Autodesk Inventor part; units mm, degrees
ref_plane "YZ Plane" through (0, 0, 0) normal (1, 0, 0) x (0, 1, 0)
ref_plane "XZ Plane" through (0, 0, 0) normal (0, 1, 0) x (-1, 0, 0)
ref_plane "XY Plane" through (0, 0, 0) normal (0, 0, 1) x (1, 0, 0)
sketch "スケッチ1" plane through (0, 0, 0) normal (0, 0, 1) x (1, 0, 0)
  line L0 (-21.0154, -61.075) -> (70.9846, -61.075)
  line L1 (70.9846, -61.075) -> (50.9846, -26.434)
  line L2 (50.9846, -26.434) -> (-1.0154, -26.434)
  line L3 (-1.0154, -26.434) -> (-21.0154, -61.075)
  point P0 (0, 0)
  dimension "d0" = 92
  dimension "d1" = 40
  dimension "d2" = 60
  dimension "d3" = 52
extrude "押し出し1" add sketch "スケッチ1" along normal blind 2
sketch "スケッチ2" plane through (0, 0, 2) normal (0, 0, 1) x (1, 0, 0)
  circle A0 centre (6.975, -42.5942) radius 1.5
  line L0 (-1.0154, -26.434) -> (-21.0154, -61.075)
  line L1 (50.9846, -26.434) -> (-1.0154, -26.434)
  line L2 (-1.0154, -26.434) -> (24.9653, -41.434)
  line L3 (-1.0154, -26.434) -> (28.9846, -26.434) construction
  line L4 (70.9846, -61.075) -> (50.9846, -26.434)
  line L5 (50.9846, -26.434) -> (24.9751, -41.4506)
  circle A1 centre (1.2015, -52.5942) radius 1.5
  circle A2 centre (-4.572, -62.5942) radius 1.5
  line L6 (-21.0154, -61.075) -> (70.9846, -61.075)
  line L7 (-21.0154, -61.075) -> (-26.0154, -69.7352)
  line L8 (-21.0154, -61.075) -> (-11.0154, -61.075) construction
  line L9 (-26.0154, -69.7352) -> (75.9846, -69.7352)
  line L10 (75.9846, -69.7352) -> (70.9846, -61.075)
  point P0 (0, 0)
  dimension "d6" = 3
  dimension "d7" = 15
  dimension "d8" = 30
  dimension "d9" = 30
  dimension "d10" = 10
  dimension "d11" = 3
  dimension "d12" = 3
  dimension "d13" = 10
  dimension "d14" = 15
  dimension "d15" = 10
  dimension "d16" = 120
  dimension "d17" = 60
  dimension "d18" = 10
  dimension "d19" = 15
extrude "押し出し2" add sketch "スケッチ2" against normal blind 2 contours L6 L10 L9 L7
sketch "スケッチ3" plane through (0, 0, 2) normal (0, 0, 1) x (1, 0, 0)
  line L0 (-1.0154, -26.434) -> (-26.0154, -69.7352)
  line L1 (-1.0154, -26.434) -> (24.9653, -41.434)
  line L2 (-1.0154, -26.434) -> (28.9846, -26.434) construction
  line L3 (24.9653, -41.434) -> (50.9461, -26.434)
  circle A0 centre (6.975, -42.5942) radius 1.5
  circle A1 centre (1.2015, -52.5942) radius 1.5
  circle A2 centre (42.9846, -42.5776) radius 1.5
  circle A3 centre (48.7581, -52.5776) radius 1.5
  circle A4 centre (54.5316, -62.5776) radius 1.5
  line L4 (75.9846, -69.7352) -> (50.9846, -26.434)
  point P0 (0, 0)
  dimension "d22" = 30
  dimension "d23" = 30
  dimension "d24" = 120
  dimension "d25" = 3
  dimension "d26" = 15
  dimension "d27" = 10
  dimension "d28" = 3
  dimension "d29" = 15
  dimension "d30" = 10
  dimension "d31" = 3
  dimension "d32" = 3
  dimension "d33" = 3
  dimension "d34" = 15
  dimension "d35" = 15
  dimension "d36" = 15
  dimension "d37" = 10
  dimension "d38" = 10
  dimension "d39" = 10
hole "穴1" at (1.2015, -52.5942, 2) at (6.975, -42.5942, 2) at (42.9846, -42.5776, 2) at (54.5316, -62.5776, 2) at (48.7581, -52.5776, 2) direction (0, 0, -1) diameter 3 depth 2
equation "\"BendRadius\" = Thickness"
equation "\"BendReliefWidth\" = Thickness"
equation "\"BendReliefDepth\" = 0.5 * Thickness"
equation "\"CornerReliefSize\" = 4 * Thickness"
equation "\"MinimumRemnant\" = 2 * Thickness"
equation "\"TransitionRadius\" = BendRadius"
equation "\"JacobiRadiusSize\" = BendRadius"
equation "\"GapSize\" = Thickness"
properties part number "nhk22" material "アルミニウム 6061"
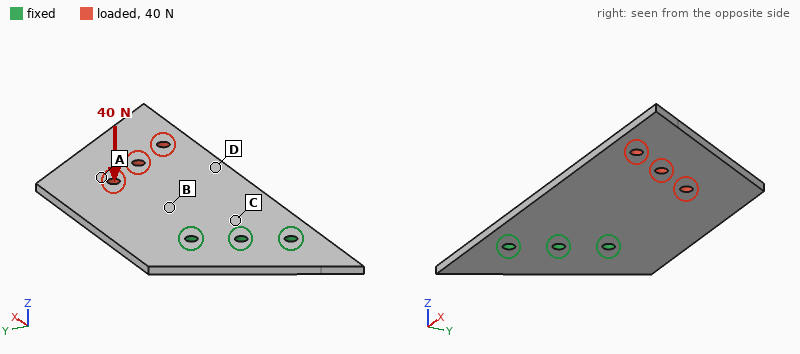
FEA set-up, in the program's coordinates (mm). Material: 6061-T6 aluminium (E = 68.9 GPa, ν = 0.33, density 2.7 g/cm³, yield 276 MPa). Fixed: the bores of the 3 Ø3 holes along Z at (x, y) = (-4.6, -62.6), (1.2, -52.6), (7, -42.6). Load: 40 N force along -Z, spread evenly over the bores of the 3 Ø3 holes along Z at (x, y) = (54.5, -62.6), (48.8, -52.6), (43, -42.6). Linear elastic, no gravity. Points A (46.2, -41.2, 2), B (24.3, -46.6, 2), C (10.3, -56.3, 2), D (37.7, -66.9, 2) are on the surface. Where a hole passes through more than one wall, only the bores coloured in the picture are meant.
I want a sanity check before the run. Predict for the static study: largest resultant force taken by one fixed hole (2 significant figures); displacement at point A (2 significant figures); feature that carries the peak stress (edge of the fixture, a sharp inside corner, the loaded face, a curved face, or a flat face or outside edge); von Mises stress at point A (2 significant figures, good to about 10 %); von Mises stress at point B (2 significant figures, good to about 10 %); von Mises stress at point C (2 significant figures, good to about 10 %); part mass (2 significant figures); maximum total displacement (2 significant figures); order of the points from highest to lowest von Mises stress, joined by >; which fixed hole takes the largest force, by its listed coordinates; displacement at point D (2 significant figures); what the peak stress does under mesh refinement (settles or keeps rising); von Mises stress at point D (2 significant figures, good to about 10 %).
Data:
50 N
0.49 mm
edge of the fixture
8.5 MPa
30 MPa
43 MPa
18 g
1.2 mm
C > B > D > A
(7, -42.6)
0.41 mm
keeps rising
18 MPa
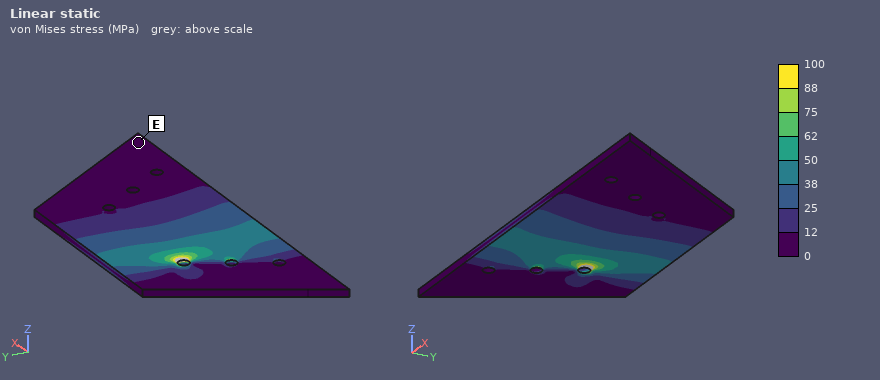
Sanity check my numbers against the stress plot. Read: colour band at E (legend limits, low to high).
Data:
0 to 12 MPa
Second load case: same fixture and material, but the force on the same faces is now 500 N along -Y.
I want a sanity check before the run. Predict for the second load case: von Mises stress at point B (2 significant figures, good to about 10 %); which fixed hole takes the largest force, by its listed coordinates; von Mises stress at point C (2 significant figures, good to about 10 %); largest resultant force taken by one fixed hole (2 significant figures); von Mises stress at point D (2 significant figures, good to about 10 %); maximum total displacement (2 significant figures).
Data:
17 MPa
(7, -42.6)
21 MPa
1.1 kN
9.8 MPa
78 µm
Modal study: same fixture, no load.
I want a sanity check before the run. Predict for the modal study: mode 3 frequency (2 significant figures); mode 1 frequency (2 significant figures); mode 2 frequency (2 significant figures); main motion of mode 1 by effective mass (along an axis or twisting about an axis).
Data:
2400 Hz
450 Hz
1400 Hz
along Z
